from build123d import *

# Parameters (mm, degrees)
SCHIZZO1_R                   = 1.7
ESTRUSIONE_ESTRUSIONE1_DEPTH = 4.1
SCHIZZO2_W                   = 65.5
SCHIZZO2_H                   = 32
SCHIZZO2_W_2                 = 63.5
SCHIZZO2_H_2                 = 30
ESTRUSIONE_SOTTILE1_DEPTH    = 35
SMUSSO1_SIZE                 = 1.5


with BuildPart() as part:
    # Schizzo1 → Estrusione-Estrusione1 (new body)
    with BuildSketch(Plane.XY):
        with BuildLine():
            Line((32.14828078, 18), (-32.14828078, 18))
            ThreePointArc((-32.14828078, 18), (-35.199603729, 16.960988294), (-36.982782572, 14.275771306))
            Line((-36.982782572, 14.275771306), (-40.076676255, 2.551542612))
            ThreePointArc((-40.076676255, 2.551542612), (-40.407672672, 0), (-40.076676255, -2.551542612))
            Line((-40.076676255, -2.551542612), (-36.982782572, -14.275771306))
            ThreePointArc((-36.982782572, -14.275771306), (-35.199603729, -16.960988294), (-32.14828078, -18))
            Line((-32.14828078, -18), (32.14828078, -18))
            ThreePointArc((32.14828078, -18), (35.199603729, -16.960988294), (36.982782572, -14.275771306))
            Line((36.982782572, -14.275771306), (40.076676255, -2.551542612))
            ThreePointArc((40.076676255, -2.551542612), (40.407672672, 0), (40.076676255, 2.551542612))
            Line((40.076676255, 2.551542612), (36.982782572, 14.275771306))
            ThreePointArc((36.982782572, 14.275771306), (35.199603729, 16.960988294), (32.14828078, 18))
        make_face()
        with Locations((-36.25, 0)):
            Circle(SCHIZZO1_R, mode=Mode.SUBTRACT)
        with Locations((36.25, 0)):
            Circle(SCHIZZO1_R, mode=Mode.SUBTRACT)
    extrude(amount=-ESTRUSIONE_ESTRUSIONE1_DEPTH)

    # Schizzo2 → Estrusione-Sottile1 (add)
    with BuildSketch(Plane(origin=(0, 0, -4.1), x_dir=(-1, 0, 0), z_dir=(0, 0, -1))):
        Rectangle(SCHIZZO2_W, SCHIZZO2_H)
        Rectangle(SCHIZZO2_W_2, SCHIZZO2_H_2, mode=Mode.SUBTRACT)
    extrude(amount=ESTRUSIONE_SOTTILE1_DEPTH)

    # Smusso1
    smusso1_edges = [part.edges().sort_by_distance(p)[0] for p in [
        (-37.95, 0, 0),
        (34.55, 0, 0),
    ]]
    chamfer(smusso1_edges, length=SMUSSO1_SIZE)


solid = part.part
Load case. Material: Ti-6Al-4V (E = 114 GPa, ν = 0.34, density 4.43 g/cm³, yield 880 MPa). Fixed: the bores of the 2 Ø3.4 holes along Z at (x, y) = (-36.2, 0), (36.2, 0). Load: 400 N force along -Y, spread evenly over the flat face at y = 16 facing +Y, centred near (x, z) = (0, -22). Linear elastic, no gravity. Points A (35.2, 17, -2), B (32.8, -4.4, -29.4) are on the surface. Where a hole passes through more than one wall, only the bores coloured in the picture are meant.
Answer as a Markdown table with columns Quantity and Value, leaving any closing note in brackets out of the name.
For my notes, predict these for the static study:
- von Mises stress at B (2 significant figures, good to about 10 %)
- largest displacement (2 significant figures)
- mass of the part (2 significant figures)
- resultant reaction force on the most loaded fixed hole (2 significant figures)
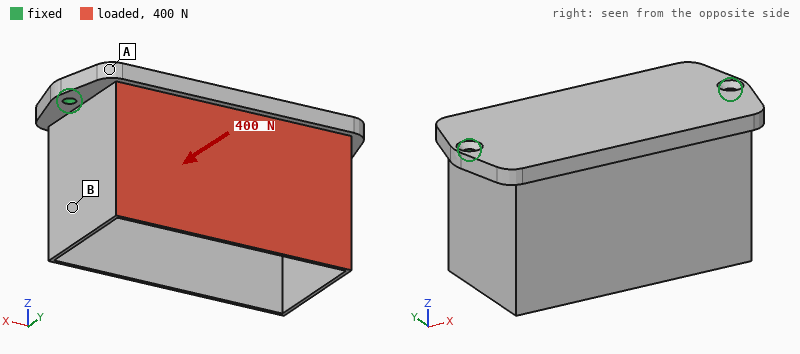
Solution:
| Quantity | Value |
|---|---|
| von Mises stress at B | 28 MPa |
| largest displacement | 0.94 mm |
| mass of the part | 79 g |
| resultant reaction force on the most loaded fixed hole | 200 N |
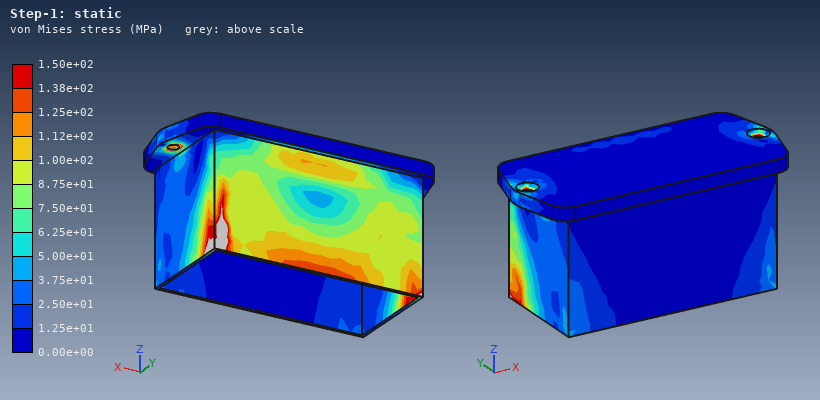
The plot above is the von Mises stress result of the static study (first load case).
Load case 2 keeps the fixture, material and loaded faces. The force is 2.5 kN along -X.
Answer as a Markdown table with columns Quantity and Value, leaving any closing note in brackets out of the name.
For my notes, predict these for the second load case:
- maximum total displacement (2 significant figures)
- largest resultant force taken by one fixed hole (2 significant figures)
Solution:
| Quantity | Value |
|---|---|
| maximum total displacement | 0.16 mm |
| largest resultant force taken by one fixed hole | 1.5 kN |
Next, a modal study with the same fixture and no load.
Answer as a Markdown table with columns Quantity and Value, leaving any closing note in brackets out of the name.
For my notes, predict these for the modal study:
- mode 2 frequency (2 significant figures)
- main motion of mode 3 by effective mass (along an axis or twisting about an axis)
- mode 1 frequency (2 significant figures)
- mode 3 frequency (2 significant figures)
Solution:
| Quantity | Value |
|---|---|
| mode 2 frequency | 1400 Hz |
| main motion of mode 3 by effective mass | twisting about X |
| mode 1 frequency | 1400 Hz |
| mode 3 frequency | 2600 Hz |
